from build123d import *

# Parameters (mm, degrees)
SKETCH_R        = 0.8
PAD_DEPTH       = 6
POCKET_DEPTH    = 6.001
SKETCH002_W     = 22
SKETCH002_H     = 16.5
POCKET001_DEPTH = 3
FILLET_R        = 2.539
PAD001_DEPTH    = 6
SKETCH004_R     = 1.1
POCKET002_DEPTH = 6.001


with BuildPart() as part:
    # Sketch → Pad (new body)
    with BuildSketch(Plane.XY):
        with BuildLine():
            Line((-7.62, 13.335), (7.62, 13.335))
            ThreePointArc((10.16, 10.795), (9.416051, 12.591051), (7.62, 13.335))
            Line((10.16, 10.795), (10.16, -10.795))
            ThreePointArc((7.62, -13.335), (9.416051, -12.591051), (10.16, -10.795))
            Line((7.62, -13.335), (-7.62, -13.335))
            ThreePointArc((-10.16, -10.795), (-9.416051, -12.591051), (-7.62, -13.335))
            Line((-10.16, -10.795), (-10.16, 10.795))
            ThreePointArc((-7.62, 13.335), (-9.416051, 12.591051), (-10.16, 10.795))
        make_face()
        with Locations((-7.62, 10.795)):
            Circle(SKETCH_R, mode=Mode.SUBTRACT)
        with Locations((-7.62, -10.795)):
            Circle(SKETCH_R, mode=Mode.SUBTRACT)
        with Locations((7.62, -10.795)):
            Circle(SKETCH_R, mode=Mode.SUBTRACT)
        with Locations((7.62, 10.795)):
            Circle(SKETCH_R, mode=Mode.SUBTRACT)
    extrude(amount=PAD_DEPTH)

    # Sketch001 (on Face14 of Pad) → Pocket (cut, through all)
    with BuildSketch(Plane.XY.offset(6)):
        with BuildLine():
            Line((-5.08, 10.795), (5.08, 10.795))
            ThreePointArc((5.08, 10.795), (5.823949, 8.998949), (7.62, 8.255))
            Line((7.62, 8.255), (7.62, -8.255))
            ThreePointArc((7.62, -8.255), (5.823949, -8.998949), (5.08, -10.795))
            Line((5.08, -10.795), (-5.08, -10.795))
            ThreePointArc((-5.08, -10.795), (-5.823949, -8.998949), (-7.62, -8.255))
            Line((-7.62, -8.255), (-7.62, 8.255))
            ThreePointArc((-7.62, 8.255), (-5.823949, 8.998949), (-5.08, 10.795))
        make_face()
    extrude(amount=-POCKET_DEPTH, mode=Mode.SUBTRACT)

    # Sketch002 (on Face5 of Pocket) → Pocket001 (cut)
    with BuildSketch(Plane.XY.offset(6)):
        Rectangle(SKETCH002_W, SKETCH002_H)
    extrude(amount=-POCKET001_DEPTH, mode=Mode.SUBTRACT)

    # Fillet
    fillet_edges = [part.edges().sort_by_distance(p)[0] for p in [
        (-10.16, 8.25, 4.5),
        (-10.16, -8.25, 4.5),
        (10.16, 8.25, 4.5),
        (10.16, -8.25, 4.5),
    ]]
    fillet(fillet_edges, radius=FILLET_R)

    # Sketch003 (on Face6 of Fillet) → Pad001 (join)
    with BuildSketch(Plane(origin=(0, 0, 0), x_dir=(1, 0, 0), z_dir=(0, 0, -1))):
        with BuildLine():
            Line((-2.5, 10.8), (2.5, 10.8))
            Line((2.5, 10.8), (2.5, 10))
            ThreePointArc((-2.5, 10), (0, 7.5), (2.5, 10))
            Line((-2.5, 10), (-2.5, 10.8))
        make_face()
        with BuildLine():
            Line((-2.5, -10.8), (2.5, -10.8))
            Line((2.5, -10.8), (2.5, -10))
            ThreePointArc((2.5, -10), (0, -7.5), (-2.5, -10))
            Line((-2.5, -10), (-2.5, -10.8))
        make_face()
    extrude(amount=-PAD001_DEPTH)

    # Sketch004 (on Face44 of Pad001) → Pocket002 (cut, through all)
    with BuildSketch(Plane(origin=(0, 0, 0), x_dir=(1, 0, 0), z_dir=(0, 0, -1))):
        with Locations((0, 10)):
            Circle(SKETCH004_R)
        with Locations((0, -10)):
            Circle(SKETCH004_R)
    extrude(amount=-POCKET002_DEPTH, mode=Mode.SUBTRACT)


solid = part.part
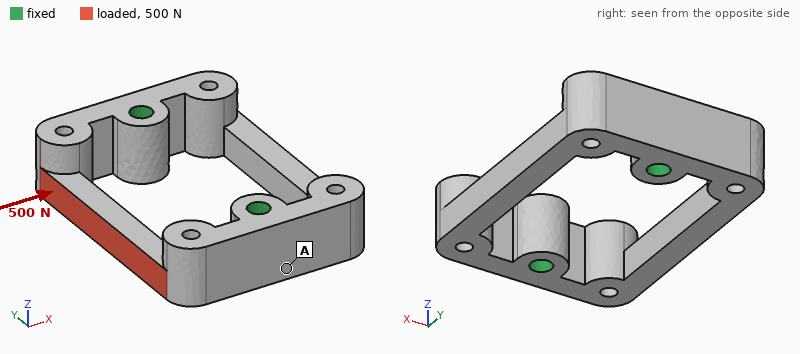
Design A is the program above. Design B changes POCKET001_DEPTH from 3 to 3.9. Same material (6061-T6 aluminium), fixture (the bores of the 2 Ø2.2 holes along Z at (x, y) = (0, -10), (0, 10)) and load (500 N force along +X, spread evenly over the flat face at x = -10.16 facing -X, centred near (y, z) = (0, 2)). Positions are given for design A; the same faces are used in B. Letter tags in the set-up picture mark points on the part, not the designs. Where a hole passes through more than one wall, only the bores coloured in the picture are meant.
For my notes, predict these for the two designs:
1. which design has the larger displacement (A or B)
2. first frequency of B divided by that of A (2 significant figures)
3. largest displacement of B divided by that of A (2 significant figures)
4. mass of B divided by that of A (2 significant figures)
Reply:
B
1.0
1.3
0.93
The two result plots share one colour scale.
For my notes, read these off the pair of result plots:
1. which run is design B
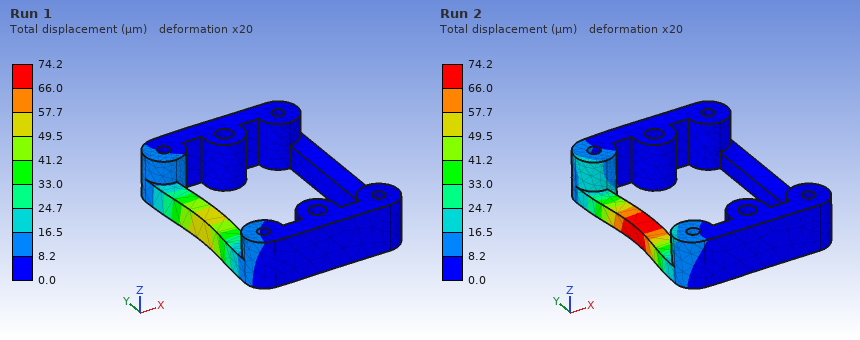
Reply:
Run 2
